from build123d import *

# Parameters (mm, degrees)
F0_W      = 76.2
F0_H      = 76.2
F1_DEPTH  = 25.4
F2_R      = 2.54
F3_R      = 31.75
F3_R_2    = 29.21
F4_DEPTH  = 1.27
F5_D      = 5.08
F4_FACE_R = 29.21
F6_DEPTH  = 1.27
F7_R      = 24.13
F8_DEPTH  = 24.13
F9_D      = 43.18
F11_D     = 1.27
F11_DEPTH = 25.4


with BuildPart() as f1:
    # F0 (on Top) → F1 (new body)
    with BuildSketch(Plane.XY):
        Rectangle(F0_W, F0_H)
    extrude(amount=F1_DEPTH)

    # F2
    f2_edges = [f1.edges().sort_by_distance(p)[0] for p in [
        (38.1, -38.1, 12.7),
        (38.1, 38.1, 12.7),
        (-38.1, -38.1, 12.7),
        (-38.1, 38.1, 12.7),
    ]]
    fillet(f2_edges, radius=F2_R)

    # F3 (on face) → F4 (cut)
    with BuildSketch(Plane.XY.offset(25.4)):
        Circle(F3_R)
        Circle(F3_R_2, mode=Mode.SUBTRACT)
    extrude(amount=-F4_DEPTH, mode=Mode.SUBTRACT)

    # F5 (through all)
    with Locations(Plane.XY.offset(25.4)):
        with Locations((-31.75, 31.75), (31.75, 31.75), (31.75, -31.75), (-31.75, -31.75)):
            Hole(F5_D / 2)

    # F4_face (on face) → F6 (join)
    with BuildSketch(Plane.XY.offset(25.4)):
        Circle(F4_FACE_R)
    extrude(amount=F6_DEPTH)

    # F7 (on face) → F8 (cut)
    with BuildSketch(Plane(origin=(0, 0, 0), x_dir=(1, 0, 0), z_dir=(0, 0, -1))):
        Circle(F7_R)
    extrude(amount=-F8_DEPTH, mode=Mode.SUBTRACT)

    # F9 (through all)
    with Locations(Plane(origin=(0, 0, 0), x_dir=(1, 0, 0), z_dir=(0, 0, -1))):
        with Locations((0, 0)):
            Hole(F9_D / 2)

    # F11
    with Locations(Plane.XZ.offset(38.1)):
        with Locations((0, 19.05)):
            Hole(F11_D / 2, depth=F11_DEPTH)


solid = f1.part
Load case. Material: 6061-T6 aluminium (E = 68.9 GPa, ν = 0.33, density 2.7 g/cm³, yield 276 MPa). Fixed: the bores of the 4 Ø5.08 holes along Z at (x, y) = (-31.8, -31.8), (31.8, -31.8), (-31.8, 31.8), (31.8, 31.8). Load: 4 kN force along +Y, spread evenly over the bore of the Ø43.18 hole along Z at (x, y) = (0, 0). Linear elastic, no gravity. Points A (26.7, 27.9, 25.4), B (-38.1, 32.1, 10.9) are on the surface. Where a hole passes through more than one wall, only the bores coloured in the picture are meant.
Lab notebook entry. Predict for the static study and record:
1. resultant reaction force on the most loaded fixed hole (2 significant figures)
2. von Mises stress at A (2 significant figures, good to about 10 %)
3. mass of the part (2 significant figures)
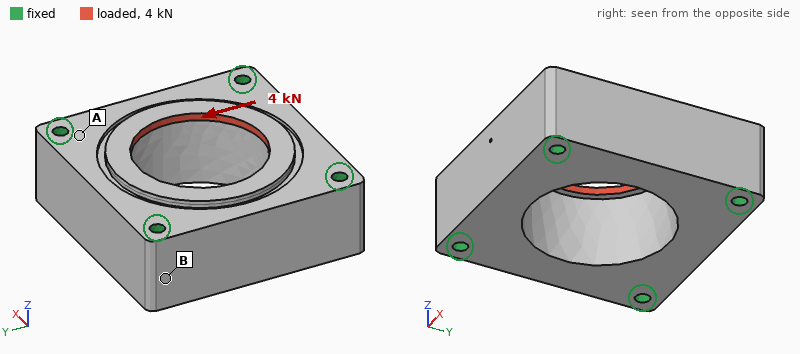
1.1 kN
5.5 MPa
270 g
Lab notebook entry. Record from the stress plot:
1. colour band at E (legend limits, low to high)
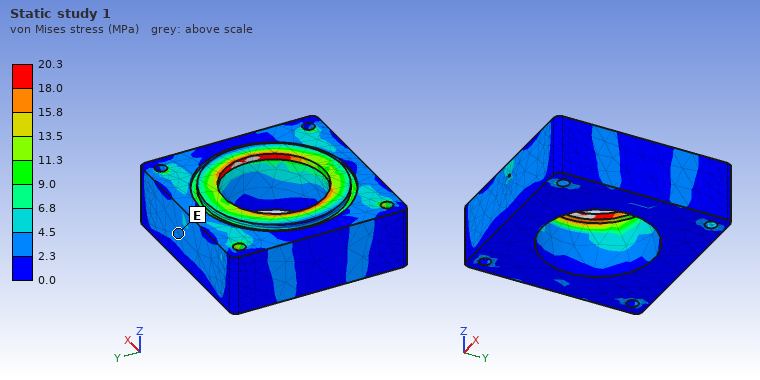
2.3 to 4.5 MPa
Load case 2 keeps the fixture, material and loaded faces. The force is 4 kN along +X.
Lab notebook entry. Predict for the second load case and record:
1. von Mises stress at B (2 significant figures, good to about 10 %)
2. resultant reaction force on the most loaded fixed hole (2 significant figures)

2.4 MPa
1.1 kN
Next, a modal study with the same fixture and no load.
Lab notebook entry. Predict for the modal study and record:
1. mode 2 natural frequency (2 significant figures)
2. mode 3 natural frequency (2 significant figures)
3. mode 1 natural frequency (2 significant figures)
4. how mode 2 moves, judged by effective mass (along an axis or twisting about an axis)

17 kHz
18 kHz
11 kHz
along Z
